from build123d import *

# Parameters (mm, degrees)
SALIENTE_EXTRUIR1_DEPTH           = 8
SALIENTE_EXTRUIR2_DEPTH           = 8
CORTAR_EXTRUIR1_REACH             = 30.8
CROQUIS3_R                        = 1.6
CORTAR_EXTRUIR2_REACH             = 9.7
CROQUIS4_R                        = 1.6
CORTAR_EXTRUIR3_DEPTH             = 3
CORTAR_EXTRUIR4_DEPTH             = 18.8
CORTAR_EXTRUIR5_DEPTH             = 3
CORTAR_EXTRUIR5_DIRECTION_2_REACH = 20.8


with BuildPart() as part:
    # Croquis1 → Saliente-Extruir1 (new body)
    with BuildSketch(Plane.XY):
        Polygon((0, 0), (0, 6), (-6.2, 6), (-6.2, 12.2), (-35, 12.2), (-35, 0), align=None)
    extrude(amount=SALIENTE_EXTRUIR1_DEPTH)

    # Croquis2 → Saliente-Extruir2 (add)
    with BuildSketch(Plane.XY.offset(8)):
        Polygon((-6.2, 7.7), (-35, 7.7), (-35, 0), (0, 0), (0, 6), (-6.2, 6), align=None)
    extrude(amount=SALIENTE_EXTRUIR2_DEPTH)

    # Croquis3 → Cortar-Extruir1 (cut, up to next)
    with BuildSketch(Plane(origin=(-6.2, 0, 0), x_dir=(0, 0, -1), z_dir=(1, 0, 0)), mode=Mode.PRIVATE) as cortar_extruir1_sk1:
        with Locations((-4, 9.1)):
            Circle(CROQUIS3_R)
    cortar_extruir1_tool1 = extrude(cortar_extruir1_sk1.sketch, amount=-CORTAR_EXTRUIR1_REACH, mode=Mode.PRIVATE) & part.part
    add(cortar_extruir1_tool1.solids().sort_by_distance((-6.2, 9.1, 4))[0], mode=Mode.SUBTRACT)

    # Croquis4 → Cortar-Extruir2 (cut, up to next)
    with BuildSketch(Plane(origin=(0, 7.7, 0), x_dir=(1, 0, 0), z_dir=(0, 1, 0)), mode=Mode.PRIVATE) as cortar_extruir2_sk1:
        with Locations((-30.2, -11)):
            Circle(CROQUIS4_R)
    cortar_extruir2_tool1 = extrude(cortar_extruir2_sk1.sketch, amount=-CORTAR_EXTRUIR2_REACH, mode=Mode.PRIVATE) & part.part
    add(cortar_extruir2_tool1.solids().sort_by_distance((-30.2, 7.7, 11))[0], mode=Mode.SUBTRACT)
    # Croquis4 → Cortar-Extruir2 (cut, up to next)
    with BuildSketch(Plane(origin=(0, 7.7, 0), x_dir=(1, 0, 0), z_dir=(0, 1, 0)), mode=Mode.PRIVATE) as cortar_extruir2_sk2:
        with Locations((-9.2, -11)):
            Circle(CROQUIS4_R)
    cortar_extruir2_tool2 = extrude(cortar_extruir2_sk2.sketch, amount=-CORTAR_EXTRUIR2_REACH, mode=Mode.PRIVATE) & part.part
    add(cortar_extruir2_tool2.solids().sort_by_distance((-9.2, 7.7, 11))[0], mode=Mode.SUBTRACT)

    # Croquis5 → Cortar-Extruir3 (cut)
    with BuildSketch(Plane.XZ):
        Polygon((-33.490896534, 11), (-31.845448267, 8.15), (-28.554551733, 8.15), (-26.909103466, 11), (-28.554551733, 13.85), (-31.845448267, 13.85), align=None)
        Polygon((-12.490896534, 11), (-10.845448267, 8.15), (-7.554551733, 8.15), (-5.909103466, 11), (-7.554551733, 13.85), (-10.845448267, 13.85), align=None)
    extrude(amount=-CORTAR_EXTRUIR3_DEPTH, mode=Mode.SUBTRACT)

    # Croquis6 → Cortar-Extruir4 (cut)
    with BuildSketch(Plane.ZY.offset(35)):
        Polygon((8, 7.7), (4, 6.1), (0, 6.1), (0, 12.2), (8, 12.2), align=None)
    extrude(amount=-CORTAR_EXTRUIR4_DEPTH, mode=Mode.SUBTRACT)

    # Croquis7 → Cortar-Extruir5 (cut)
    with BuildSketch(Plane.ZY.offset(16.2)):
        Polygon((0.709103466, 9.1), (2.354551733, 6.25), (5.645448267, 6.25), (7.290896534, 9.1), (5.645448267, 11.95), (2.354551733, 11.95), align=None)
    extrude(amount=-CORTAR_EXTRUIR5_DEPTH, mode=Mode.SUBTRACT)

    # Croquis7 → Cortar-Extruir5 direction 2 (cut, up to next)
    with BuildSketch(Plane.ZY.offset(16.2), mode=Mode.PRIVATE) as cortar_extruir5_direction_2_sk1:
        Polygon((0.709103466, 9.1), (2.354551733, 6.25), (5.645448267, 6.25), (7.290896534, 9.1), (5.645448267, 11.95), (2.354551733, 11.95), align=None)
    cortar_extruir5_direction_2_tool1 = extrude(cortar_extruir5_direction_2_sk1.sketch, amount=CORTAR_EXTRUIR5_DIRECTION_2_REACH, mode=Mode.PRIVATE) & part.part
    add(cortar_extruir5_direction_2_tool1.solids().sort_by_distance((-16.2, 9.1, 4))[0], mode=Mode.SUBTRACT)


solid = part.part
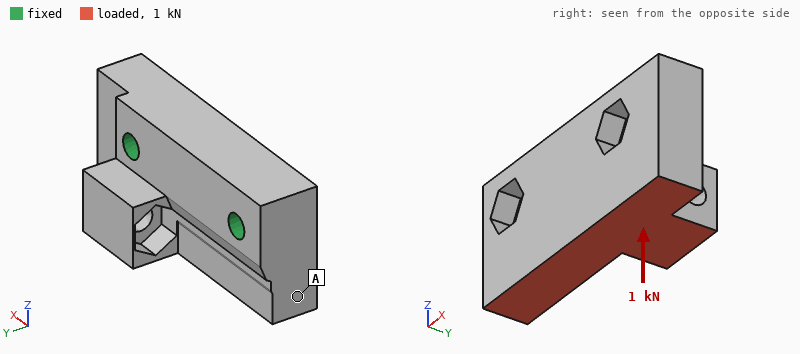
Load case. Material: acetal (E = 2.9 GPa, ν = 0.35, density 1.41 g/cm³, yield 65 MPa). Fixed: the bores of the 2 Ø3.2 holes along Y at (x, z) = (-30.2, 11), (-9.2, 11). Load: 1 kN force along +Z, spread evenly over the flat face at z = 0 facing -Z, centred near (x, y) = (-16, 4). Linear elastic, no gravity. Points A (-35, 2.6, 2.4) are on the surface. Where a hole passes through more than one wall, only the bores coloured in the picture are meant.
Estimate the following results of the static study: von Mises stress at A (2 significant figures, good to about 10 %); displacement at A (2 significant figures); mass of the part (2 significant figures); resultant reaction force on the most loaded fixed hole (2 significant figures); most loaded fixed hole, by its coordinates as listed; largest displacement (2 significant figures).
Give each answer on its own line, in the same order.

3.6 MPa
0.042 mm
5.5 g
670 N
(-9.2, 11)
0.10 mm
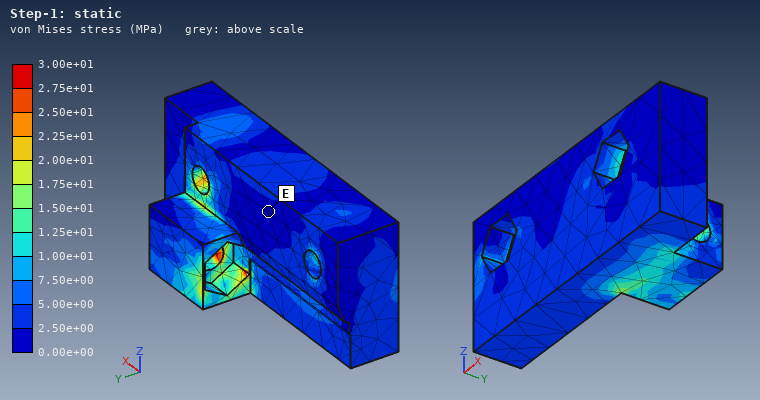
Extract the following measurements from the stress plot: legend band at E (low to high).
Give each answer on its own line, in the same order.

0.00e+00 to 2.50e+00 MPa
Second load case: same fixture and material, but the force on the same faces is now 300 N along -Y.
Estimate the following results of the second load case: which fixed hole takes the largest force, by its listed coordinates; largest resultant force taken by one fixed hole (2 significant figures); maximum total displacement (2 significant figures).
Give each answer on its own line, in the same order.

(-9.2, 11)
200 N
0.22 mm
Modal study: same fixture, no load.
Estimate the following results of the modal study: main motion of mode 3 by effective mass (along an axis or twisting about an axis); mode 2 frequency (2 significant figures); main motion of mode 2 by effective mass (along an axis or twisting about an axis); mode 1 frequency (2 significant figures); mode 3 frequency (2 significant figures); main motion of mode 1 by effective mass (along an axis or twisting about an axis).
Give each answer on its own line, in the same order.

along X
7800 Hz
twisting about Z
5500 Hz
10 kHz
along Y
